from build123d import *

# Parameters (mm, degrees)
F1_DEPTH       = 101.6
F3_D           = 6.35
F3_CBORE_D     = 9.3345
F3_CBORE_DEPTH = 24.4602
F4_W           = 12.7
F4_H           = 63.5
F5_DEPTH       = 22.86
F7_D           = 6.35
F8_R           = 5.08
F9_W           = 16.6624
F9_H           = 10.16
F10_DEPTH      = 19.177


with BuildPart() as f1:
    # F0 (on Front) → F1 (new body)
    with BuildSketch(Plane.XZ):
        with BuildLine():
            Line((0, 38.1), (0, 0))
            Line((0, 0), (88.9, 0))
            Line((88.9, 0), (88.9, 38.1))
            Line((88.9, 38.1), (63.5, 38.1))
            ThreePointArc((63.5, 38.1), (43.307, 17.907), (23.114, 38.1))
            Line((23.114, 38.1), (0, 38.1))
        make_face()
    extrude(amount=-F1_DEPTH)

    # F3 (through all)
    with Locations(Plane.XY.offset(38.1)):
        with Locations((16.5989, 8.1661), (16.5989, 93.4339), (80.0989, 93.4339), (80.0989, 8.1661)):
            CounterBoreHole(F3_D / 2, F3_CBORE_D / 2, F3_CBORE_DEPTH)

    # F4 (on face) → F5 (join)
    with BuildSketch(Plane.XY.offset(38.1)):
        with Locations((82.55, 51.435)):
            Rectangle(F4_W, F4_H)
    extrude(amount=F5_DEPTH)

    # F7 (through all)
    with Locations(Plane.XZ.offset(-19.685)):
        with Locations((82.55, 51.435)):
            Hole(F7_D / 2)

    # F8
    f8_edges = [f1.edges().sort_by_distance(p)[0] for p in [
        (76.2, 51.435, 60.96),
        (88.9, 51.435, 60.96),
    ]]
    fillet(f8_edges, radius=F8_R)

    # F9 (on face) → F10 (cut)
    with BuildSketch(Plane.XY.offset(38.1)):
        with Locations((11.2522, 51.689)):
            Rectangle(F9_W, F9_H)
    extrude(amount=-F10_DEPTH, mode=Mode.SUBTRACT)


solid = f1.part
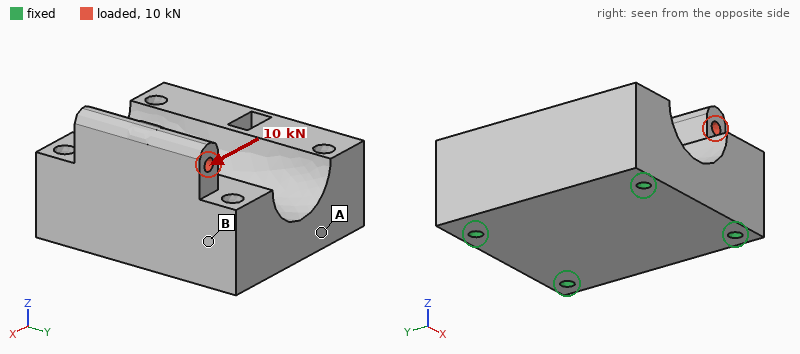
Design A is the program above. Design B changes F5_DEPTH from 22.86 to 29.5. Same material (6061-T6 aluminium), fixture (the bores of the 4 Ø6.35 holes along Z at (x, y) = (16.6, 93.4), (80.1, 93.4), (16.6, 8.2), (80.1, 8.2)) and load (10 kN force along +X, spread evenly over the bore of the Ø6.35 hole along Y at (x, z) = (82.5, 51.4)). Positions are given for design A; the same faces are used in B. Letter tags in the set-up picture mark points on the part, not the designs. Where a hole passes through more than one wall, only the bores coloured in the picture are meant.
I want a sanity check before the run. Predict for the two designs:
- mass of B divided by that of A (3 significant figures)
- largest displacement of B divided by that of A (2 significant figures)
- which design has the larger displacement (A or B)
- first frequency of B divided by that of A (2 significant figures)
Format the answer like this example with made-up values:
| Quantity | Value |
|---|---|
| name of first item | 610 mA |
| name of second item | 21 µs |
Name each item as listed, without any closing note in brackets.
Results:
| Quantity | Value |
|---|---|
| mass of B divided by that of A | 1.02 |
| largest displacement of B divided by that of A | 1.2 |
| which design has the larger displacement | B |
| first frequency of B divided by that of A | 0.82 |
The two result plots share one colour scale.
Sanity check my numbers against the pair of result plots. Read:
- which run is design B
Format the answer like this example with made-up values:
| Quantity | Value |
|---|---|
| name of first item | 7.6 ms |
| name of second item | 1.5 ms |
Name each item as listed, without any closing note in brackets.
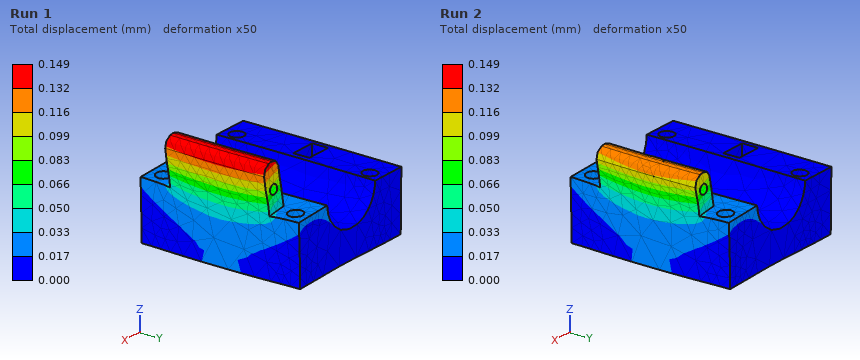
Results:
| Quantity | Value |
|---|---|
| which run is design B | Run 1 |
